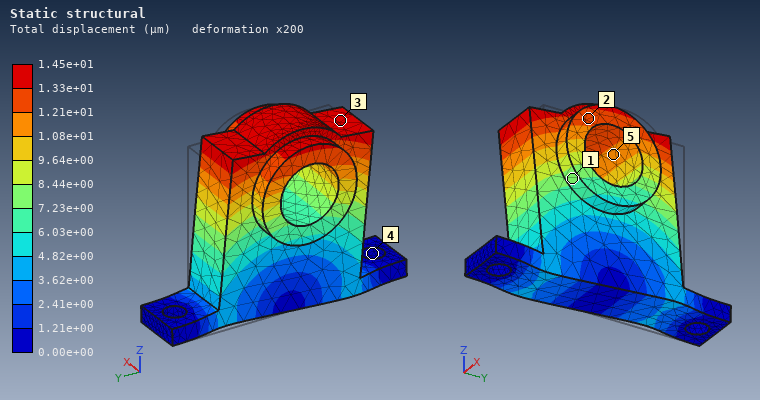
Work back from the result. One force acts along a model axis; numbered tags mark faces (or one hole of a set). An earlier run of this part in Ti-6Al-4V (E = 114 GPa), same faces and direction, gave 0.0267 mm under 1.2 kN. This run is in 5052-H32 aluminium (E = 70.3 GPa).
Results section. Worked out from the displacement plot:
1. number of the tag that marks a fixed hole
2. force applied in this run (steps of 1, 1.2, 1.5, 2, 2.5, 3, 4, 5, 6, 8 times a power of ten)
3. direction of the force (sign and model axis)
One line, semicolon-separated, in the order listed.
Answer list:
4; 400 N; -Y
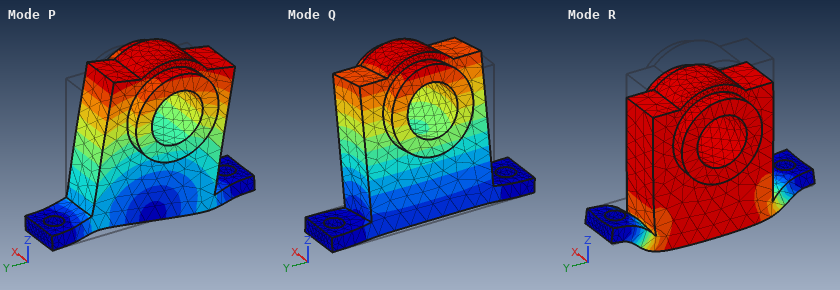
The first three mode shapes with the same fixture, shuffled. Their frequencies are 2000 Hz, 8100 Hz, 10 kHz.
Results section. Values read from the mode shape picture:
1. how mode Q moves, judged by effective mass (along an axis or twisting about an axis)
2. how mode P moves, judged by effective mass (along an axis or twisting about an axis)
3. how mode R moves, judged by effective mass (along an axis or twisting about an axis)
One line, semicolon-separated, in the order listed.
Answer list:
along X; along Y; along Z
